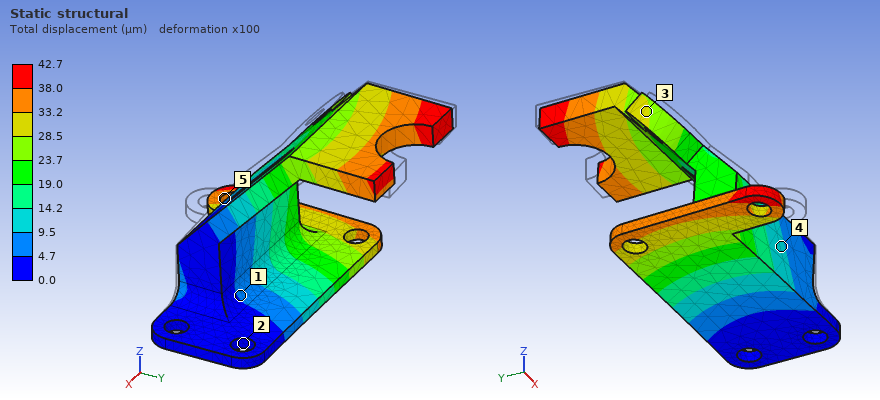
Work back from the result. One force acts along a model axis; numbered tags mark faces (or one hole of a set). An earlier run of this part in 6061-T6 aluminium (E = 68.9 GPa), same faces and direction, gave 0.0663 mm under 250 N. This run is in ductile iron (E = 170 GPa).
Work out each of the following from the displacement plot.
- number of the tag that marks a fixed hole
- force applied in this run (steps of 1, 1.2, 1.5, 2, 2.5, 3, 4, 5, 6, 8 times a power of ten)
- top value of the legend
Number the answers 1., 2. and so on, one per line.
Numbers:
1. 2
2. 400 N
3. 42.7 µm
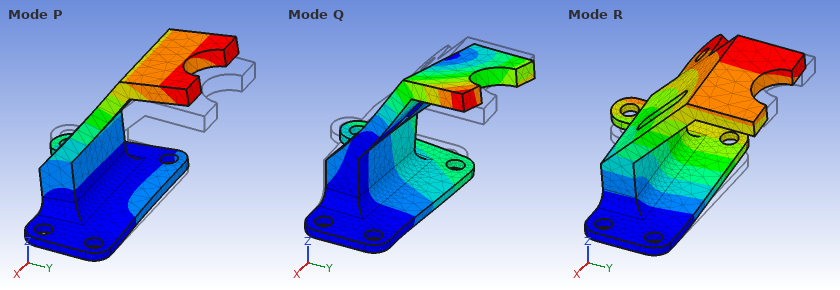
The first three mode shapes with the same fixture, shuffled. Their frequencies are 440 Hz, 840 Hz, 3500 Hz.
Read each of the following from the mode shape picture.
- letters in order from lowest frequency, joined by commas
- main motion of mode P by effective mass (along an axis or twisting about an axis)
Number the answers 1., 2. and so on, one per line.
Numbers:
1. R, P, Q
2. along Y
